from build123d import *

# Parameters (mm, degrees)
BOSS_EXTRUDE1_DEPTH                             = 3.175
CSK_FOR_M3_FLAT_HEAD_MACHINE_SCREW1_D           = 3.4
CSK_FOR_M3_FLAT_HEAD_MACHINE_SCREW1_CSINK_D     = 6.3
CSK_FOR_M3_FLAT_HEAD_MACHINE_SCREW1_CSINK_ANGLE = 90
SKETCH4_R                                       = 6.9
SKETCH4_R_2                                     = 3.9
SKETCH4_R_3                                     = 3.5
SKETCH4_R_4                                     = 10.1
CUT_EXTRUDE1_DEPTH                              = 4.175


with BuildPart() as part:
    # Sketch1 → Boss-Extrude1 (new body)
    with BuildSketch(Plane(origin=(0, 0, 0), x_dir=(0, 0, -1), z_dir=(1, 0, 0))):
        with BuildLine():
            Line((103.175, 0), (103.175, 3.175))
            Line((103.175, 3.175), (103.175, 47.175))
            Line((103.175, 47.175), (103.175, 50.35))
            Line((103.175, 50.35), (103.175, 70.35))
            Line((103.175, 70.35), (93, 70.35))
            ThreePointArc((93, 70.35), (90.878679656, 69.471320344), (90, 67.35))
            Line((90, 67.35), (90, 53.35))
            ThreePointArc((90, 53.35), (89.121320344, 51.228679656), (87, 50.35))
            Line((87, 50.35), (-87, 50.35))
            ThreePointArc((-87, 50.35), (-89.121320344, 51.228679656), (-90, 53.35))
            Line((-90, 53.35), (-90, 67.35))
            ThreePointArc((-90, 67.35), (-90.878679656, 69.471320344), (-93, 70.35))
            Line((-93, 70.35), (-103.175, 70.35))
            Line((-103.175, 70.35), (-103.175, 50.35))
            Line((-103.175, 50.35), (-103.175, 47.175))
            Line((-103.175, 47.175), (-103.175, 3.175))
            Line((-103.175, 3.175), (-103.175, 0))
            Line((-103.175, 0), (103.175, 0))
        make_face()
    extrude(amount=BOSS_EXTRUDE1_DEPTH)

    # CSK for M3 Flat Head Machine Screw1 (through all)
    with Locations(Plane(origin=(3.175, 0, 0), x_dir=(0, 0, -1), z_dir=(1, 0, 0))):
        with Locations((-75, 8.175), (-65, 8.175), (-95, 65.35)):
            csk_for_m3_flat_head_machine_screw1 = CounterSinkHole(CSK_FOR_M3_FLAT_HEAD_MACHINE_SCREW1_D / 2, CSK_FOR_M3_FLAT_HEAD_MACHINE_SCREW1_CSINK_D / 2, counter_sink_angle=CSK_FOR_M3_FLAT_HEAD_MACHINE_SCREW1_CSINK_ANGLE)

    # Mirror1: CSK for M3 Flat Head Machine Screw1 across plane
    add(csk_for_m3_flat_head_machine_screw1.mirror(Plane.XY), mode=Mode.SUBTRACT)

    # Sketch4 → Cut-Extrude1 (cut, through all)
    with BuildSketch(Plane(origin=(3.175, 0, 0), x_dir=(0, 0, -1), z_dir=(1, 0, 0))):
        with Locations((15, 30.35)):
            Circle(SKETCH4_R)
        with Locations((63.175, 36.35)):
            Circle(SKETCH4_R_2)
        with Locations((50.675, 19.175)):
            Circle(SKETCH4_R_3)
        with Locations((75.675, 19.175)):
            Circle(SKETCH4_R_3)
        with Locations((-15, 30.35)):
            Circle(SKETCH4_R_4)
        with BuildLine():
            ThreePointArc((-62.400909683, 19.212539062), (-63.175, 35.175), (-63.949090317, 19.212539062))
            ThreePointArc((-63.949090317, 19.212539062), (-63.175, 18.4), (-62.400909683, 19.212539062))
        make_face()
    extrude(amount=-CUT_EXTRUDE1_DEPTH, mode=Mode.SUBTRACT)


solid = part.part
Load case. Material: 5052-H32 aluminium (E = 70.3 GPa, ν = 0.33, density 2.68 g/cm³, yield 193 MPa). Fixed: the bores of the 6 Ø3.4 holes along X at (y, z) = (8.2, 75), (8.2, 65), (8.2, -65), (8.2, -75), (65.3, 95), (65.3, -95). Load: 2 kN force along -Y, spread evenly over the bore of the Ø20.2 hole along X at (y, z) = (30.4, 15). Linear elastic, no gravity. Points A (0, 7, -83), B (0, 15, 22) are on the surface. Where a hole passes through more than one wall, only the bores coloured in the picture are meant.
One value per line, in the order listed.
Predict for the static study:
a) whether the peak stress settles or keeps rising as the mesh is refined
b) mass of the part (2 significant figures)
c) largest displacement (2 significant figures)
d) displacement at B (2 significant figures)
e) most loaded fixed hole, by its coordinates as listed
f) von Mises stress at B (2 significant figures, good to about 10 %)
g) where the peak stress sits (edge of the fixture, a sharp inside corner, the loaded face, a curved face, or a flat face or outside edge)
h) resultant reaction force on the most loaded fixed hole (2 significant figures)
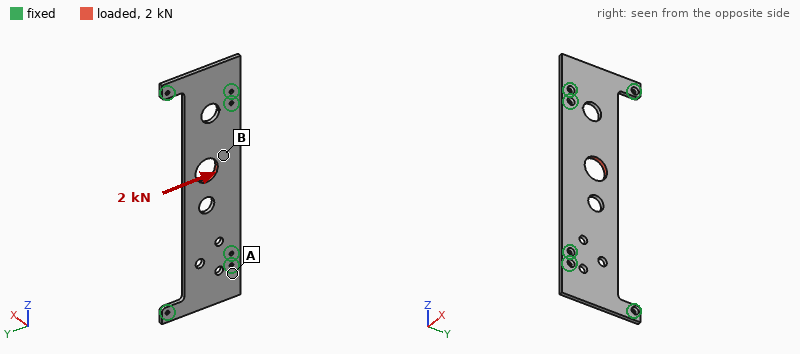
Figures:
keeps rising
85 g
50 µm
40 µm
(8.2, 65)
13 MPa
edge of the fixture
1.4 kN
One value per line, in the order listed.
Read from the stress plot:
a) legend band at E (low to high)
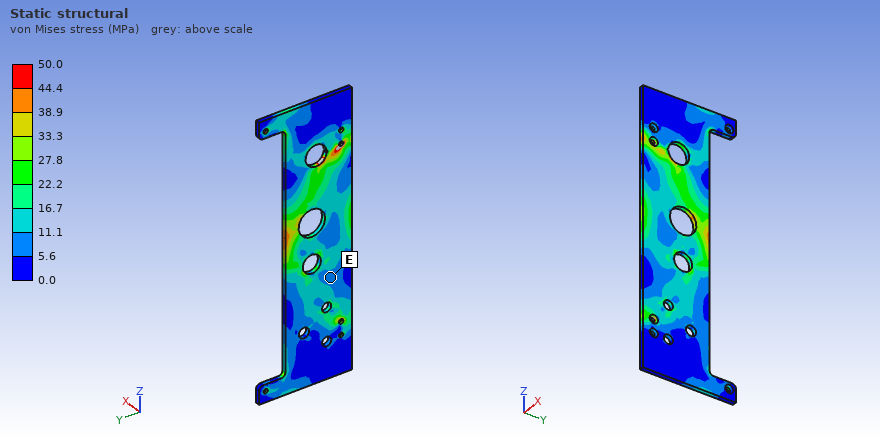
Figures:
5.6 to 11.1 MPa
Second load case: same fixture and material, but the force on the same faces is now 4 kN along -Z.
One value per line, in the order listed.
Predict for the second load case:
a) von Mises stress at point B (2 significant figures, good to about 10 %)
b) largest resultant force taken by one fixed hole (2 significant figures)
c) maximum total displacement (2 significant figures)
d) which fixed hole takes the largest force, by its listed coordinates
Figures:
21 MPa
1.3 kN
26 µm
(8.2, 65)
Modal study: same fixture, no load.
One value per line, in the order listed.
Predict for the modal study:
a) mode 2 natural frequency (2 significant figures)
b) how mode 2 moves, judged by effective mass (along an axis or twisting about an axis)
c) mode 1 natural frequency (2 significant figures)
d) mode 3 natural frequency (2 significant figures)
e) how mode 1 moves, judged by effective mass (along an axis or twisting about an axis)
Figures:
1400 Hz
twisting about Z
690 Hz
1700 Hz
along X
